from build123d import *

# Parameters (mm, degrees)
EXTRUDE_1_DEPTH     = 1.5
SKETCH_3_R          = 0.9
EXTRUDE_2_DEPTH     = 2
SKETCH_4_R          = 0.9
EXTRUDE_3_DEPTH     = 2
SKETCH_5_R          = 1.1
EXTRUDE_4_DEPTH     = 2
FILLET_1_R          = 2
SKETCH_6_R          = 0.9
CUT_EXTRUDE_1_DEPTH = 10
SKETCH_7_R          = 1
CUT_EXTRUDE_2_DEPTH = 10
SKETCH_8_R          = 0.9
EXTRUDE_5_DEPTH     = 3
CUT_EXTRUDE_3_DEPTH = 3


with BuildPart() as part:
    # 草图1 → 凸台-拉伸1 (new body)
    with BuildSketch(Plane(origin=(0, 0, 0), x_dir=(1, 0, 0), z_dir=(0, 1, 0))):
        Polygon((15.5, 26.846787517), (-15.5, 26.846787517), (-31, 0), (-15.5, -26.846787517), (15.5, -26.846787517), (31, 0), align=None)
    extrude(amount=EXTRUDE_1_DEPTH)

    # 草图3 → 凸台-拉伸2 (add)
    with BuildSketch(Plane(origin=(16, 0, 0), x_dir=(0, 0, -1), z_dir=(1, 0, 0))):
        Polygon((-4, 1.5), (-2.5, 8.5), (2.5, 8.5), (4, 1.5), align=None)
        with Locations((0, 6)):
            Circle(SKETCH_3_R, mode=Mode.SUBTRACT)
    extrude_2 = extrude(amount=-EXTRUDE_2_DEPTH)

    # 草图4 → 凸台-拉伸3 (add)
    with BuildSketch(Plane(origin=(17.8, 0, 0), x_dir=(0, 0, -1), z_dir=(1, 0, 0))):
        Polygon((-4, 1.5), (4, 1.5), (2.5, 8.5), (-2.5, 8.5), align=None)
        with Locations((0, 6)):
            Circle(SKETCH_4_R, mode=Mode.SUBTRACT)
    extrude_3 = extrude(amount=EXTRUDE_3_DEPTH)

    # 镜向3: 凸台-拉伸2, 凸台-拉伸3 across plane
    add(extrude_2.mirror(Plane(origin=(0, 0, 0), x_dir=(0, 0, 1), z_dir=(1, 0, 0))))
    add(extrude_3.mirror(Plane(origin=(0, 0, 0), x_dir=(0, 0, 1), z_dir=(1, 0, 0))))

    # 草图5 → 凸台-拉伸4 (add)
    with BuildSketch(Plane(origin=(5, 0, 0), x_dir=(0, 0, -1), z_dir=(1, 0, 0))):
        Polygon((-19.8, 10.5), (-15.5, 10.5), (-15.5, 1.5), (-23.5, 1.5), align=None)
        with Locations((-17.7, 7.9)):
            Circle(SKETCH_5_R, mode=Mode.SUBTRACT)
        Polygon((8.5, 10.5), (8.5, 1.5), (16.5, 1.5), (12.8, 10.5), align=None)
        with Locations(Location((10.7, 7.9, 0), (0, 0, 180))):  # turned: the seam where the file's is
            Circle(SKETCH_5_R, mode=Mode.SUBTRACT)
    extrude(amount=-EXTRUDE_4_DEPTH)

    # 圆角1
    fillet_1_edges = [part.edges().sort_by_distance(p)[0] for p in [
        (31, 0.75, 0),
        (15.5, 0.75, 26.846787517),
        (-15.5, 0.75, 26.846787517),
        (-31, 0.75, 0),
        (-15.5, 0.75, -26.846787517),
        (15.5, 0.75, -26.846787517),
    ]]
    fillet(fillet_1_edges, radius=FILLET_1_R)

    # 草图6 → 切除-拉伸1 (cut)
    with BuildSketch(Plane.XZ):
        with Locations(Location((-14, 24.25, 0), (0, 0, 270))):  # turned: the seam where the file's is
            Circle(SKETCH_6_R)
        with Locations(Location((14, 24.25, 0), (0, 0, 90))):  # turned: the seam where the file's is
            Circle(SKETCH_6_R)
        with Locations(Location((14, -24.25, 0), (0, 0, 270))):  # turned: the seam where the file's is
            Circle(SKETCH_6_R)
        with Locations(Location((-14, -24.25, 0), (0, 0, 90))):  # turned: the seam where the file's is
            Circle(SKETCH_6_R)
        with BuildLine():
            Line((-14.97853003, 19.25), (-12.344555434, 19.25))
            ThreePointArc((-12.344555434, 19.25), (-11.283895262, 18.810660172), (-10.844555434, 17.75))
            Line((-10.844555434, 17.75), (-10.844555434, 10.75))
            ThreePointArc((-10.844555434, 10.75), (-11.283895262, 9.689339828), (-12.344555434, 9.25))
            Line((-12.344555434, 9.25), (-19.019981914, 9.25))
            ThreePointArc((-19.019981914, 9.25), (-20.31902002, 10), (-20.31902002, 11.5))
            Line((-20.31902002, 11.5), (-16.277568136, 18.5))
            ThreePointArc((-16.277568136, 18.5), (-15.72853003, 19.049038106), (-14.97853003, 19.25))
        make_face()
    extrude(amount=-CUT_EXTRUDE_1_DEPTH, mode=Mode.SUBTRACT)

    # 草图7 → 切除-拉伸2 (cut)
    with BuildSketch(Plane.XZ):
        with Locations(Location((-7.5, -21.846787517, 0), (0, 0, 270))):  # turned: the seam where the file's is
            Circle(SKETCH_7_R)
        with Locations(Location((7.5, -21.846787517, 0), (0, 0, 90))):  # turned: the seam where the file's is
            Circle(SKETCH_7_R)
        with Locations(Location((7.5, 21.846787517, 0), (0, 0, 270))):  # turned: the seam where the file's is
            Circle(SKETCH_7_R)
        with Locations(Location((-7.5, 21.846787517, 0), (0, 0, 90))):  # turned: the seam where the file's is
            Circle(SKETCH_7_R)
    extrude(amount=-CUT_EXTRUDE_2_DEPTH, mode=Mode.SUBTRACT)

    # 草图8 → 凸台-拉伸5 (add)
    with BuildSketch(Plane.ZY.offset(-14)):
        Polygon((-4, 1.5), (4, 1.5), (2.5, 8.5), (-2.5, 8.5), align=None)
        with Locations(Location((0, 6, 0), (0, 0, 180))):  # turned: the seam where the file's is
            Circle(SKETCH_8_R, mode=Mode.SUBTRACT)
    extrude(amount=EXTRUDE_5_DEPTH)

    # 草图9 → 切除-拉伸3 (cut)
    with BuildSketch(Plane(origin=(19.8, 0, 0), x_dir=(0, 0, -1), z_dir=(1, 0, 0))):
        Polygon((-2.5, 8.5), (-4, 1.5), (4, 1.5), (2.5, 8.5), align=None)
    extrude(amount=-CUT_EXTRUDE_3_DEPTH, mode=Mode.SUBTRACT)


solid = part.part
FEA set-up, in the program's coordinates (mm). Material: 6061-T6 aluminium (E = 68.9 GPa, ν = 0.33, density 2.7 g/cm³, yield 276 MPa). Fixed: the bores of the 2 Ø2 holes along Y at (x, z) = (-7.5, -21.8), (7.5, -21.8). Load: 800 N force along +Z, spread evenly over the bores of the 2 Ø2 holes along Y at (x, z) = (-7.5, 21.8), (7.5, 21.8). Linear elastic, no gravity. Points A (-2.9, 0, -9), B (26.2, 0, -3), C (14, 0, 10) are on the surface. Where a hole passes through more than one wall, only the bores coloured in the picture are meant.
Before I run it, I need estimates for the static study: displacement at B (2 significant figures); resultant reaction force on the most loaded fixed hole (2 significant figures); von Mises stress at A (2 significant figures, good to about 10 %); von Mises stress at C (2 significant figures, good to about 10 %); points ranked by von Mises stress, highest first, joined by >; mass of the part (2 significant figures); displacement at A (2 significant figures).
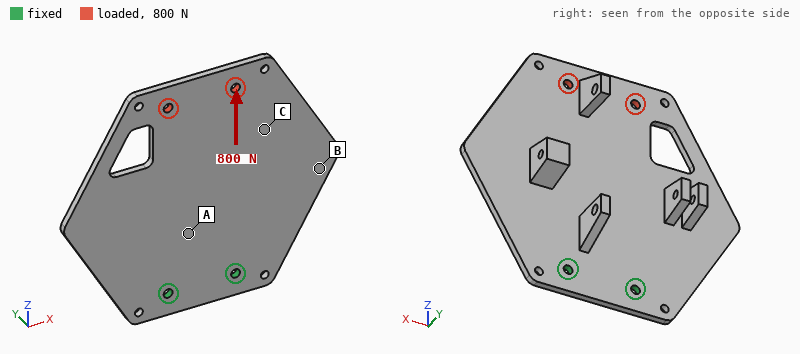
6.4 µm
400 N
19 MPa
11 MPa
A > C > B
11 g
4.4 µm
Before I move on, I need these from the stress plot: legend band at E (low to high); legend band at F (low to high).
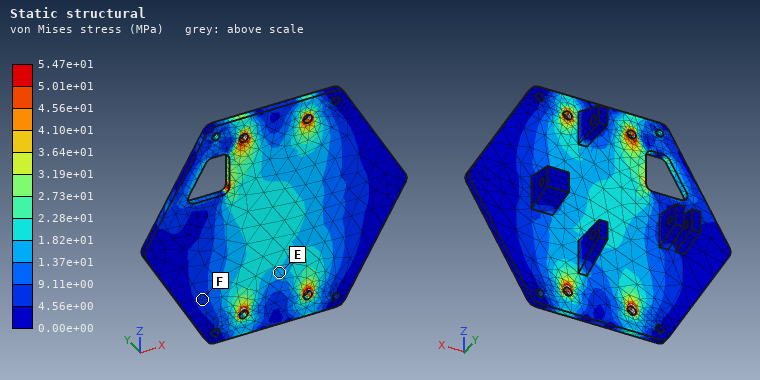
1.37e+01 to 1.82e+01 MPa
4.56e+00 to 9.11e+00 MPa
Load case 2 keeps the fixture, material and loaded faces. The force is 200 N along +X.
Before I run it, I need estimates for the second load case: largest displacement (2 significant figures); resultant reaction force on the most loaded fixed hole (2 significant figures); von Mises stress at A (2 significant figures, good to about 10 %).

49 µm
550 N
18 MPa
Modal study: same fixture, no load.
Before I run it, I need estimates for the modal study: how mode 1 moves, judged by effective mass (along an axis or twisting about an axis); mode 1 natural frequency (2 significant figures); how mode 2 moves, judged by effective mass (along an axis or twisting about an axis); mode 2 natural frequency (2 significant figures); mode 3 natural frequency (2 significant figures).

along Y
510 Hz
twisting about Z
1100 Hz
2300 Hz
